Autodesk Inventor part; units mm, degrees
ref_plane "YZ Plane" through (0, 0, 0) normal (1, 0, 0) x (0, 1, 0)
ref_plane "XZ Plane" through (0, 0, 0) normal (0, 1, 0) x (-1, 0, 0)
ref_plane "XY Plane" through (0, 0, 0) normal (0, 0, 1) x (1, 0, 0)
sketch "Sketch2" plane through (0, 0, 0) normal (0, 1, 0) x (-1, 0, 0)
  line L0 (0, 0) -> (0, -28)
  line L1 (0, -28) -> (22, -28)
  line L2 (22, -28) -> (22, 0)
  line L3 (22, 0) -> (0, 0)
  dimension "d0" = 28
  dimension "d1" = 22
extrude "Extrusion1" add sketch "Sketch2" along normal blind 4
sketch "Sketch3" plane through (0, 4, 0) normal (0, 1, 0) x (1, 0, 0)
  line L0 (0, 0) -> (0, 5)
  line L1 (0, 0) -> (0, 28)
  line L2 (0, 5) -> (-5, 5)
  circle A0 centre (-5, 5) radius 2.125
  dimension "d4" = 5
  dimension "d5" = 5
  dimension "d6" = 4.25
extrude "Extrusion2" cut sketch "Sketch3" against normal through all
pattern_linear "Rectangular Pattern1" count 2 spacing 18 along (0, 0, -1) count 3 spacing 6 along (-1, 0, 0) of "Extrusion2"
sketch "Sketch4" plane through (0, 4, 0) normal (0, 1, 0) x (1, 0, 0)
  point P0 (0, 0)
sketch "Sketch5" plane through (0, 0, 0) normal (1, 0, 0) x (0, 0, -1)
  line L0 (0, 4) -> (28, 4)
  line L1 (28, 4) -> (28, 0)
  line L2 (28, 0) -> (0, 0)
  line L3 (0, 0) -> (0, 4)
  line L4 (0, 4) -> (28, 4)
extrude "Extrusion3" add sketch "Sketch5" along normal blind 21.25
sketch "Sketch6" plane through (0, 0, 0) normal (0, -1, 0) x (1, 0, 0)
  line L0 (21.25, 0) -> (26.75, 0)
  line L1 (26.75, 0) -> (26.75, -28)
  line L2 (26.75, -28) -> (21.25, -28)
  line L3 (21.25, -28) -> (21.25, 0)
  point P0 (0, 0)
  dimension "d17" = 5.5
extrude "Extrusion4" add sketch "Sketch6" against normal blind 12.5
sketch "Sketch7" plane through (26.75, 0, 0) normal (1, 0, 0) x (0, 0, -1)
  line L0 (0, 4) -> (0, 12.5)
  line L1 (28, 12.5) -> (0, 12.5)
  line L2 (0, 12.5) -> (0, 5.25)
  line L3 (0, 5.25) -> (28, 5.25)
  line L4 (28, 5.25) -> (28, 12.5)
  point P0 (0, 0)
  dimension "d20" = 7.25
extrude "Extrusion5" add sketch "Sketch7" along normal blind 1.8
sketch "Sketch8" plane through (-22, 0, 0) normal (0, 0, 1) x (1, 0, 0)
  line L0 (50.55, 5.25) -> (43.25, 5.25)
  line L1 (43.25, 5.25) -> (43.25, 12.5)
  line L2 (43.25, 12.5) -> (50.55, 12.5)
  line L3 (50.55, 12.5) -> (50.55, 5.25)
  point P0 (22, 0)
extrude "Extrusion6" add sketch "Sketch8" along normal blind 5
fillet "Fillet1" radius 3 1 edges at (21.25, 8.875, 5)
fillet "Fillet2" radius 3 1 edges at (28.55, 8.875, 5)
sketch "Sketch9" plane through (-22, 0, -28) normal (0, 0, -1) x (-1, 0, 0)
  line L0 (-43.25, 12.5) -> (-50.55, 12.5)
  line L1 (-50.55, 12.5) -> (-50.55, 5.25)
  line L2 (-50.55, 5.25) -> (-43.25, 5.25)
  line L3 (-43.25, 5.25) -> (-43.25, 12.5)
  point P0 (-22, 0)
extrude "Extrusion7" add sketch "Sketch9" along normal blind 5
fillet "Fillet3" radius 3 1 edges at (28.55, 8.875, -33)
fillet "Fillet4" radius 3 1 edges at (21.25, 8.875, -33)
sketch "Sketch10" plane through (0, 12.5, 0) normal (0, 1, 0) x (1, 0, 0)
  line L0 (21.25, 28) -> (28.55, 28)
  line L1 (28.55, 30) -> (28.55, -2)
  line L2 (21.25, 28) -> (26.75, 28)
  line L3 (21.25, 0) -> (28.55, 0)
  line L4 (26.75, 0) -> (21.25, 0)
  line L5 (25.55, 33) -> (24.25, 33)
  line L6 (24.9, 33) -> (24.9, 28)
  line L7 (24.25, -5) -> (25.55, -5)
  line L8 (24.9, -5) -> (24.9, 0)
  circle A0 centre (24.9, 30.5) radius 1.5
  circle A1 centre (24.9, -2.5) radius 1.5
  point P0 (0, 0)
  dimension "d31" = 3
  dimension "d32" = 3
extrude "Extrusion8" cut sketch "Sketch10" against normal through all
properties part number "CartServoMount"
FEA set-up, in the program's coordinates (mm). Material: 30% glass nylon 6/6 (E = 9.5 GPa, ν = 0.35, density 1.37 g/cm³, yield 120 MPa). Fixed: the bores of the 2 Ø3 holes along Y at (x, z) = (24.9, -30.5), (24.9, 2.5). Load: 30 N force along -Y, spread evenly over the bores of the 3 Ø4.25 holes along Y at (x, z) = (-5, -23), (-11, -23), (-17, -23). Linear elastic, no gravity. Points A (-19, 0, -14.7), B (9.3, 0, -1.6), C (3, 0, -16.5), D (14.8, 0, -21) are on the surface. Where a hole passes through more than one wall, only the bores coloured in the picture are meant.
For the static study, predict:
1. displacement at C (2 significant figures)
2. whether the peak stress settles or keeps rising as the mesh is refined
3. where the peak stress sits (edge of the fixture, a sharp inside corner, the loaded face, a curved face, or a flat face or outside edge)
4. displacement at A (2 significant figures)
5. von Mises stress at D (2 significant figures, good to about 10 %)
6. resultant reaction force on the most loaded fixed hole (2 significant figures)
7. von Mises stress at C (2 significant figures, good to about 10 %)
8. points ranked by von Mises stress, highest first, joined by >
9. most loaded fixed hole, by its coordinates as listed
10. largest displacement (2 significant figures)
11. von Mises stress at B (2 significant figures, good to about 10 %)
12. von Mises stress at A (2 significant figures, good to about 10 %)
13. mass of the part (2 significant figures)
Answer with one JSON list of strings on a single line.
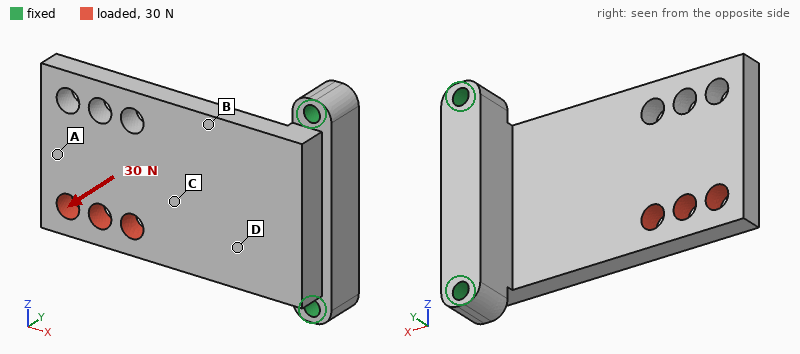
["0.19 mm", "keeps rising", "edge of the fixture", "0.51 mm", "10 MPa", "29 N", "6.3 MPa", "D > B > C > A", "(24.9, -30.5)", "0.61 mm", "8.4 MPa", "1.4 MPa", "9.8 g"]
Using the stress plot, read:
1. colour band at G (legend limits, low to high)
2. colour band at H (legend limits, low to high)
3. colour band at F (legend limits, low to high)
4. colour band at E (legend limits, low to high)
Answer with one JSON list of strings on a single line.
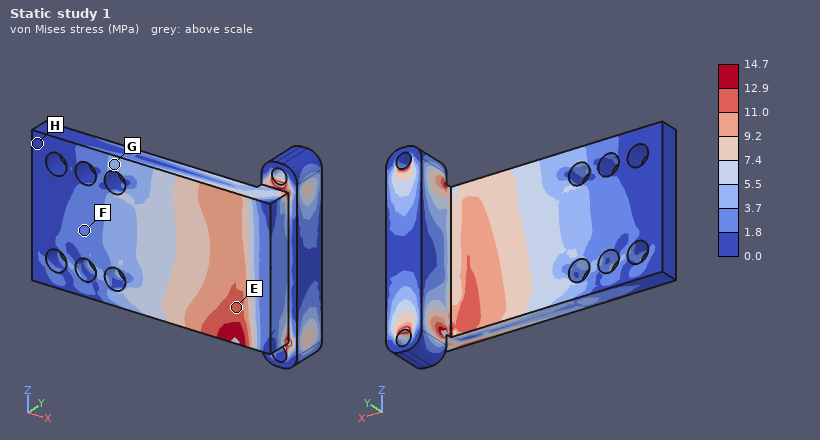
["3.7 to 5.5 MPa", "0.0 to 1.8 MPa", "1.8 to 3.7 MPa", "11.0 to 12.9 MPa"]
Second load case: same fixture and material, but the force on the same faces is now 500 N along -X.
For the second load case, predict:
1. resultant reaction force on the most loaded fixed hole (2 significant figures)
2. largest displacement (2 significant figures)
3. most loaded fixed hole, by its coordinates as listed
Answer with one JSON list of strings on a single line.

["410 N", "0.43 mm", "(24.9, -30.5)"]
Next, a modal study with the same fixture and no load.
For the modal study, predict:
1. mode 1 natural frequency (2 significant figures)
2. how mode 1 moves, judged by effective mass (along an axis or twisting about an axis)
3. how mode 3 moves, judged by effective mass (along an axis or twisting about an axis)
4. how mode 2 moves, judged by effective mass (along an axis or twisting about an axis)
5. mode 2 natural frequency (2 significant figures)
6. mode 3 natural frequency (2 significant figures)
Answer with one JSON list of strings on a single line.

["760 Hz", "along Y", "along Z", "along Z", "2600 Hz", "3200 Hz"]
